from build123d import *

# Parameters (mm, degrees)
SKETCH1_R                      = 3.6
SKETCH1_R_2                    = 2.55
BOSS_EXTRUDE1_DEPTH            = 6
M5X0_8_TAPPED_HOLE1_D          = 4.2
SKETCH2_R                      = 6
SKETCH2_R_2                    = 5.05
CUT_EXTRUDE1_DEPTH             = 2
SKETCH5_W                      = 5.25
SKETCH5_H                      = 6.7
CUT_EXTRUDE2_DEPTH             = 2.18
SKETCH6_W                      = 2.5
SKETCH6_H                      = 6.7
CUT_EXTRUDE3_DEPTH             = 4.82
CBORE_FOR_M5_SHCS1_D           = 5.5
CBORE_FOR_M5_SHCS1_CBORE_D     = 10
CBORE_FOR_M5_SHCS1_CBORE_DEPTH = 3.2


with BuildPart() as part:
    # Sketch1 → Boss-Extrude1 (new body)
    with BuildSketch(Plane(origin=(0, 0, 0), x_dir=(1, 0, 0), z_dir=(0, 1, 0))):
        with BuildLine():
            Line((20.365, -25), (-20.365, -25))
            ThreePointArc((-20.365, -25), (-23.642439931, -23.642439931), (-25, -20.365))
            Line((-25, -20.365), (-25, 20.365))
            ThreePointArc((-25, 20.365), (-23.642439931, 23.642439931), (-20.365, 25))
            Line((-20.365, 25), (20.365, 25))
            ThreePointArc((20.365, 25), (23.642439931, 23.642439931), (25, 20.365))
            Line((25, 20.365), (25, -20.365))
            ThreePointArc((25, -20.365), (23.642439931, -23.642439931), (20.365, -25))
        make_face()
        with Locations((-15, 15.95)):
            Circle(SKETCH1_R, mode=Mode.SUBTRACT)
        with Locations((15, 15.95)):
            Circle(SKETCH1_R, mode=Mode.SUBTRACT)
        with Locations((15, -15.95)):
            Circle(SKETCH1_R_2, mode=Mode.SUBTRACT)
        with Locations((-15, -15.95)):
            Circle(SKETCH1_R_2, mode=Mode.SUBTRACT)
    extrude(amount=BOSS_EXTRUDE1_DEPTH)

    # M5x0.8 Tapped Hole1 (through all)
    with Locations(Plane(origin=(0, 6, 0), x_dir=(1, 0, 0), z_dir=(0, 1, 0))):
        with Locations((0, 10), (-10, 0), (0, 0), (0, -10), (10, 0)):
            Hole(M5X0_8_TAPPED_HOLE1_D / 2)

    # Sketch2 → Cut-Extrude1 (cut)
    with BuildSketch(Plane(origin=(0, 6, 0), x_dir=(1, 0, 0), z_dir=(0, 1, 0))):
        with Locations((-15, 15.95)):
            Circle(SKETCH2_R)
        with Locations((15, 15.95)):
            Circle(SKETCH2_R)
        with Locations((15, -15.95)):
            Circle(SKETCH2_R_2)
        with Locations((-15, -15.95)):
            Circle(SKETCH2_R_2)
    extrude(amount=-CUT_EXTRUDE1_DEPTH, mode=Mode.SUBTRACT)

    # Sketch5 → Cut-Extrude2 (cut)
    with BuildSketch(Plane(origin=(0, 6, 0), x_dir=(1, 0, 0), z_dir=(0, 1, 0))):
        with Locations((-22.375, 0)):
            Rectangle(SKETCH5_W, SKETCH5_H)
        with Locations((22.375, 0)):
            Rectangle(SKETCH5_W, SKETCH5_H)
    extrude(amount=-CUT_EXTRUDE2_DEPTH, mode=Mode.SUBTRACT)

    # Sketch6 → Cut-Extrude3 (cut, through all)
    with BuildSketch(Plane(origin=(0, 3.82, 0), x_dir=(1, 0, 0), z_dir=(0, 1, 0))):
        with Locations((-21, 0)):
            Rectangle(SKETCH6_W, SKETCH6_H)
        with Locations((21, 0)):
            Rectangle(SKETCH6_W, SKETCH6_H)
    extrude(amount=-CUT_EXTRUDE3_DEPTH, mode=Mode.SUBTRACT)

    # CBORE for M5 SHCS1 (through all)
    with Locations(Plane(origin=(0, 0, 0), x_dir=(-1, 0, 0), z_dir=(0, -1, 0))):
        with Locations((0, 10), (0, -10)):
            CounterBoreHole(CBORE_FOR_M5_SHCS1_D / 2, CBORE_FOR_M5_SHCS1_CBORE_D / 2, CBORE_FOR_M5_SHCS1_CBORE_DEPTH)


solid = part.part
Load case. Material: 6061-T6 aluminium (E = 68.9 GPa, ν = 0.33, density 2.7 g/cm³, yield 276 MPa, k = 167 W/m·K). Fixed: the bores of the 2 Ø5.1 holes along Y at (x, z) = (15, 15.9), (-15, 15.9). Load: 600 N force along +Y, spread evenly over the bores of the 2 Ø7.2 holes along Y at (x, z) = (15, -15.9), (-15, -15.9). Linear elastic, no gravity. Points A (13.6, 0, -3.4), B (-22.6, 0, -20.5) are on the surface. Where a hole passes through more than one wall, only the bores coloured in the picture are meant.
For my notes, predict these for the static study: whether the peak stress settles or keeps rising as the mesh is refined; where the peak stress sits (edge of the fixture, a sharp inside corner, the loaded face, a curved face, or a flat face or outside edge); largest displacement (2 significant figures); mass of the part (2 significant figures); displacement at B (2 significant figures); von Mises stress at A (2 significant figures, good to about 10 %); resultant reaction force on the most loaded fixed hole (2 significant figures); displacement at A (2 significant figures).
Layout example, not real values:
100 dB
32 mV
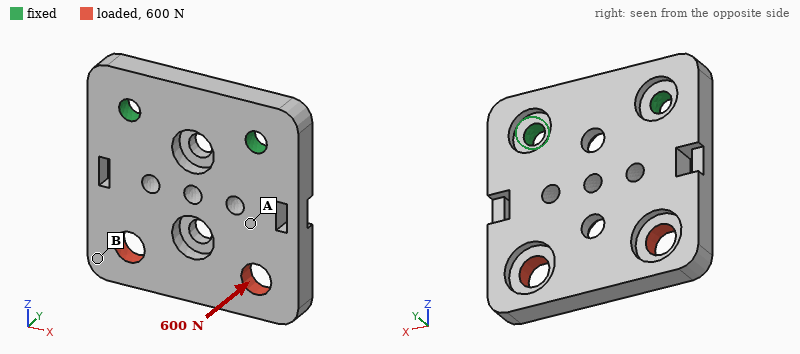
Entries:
keeps rising
edge of the fixture
0.26 mm
34 g
0.22 mm
37 MPa
310 N
0.090 mm
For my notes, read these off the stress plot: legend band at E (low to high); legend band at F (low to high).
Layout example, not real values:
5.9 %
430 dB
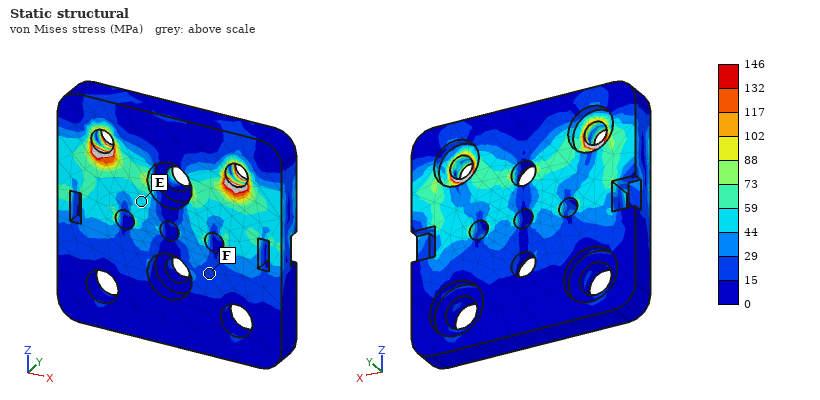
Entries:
44 to 59 MPa
15 to 29 MPa
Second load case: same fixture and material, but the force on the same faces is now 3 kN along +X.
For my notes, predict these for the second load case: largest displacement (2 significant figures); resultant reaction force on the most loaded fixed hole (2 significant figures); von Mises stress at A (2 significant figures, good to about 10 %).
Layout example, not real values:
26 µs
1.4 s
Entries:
72 µm
3.2 kN
35 MPa
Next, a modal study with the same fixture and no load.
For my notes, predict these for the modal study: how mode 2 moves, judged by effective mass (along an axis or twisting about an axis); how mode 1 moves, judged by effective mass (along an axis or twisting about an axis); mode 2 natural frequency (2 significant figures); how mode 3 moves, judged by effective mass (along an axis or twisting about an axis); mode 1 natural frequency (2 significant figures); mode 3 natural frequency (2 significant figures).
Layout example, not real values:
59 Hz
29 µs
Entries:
twisting about Z
along Y
5100 Hz
along X
2400 Hz
11 kHz
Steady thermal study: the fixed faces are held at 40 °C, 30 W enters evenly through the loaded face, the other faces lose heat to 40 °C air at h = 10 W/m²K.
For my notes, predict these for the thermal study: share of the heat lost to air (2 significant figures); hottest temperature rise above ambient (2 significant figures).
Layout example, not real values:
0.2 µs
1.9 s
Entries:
3.0 %
30 K
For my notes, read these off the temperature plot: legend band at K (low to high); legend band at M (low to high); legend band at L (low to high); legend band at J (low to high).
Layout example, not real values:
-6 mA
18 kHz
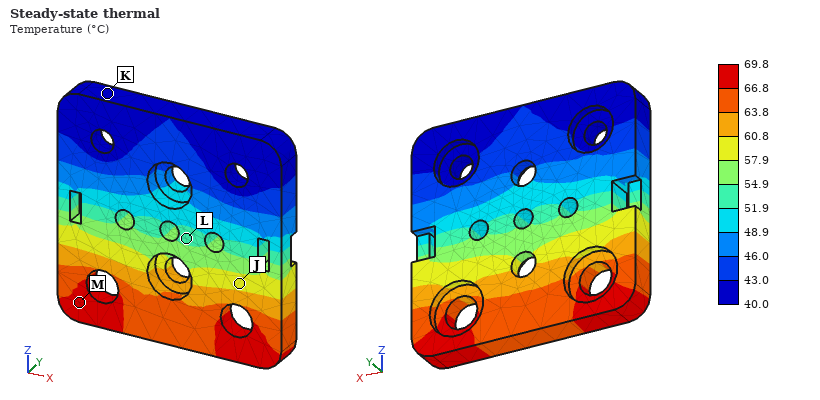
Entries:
40.0 to 43.0 °C
66.8 to 69.8 °C
51.9 to 54.9 °C
57.9 to 60.8 °C
